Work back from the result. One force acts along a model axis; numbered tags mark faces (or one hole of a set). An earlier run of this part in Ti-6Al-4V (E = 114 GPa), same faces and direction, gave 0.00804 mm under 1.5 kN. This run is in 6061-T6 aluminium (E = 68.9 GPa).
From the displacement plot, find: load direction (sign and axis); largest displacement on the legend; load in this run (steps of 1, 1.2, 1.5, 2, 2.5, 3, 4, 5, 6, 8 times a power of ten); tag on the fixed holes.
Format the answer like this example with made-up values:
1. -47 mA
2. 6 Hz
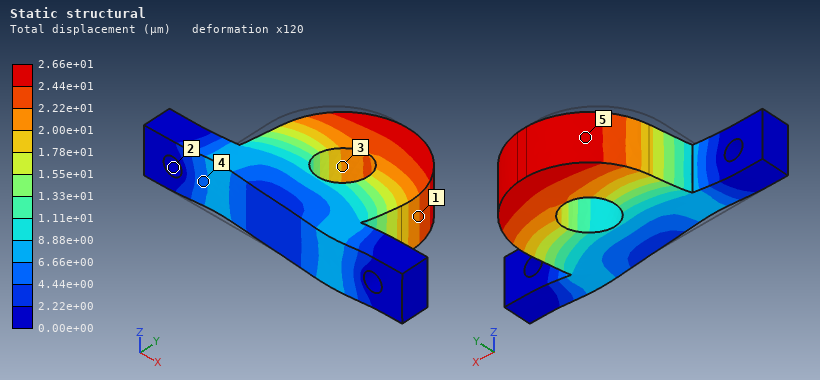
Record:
1. +X
2. 2.66e+01 µm
3. 3 kN
4. 2
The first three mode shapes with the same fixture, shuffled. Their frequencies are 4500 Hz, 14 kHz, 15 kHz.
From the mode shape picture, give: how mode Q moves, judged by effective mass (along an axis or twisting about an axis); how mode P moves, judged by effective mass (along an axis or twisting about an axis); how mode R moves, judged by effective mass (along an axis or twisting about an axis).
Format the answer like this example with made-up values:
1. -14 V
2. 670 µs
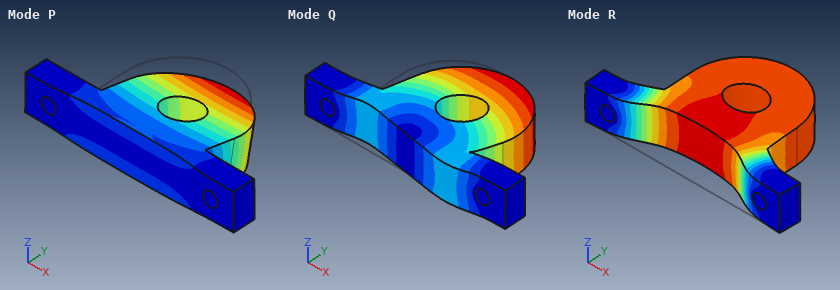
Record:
1. along X
2. along Z
3. along Y
